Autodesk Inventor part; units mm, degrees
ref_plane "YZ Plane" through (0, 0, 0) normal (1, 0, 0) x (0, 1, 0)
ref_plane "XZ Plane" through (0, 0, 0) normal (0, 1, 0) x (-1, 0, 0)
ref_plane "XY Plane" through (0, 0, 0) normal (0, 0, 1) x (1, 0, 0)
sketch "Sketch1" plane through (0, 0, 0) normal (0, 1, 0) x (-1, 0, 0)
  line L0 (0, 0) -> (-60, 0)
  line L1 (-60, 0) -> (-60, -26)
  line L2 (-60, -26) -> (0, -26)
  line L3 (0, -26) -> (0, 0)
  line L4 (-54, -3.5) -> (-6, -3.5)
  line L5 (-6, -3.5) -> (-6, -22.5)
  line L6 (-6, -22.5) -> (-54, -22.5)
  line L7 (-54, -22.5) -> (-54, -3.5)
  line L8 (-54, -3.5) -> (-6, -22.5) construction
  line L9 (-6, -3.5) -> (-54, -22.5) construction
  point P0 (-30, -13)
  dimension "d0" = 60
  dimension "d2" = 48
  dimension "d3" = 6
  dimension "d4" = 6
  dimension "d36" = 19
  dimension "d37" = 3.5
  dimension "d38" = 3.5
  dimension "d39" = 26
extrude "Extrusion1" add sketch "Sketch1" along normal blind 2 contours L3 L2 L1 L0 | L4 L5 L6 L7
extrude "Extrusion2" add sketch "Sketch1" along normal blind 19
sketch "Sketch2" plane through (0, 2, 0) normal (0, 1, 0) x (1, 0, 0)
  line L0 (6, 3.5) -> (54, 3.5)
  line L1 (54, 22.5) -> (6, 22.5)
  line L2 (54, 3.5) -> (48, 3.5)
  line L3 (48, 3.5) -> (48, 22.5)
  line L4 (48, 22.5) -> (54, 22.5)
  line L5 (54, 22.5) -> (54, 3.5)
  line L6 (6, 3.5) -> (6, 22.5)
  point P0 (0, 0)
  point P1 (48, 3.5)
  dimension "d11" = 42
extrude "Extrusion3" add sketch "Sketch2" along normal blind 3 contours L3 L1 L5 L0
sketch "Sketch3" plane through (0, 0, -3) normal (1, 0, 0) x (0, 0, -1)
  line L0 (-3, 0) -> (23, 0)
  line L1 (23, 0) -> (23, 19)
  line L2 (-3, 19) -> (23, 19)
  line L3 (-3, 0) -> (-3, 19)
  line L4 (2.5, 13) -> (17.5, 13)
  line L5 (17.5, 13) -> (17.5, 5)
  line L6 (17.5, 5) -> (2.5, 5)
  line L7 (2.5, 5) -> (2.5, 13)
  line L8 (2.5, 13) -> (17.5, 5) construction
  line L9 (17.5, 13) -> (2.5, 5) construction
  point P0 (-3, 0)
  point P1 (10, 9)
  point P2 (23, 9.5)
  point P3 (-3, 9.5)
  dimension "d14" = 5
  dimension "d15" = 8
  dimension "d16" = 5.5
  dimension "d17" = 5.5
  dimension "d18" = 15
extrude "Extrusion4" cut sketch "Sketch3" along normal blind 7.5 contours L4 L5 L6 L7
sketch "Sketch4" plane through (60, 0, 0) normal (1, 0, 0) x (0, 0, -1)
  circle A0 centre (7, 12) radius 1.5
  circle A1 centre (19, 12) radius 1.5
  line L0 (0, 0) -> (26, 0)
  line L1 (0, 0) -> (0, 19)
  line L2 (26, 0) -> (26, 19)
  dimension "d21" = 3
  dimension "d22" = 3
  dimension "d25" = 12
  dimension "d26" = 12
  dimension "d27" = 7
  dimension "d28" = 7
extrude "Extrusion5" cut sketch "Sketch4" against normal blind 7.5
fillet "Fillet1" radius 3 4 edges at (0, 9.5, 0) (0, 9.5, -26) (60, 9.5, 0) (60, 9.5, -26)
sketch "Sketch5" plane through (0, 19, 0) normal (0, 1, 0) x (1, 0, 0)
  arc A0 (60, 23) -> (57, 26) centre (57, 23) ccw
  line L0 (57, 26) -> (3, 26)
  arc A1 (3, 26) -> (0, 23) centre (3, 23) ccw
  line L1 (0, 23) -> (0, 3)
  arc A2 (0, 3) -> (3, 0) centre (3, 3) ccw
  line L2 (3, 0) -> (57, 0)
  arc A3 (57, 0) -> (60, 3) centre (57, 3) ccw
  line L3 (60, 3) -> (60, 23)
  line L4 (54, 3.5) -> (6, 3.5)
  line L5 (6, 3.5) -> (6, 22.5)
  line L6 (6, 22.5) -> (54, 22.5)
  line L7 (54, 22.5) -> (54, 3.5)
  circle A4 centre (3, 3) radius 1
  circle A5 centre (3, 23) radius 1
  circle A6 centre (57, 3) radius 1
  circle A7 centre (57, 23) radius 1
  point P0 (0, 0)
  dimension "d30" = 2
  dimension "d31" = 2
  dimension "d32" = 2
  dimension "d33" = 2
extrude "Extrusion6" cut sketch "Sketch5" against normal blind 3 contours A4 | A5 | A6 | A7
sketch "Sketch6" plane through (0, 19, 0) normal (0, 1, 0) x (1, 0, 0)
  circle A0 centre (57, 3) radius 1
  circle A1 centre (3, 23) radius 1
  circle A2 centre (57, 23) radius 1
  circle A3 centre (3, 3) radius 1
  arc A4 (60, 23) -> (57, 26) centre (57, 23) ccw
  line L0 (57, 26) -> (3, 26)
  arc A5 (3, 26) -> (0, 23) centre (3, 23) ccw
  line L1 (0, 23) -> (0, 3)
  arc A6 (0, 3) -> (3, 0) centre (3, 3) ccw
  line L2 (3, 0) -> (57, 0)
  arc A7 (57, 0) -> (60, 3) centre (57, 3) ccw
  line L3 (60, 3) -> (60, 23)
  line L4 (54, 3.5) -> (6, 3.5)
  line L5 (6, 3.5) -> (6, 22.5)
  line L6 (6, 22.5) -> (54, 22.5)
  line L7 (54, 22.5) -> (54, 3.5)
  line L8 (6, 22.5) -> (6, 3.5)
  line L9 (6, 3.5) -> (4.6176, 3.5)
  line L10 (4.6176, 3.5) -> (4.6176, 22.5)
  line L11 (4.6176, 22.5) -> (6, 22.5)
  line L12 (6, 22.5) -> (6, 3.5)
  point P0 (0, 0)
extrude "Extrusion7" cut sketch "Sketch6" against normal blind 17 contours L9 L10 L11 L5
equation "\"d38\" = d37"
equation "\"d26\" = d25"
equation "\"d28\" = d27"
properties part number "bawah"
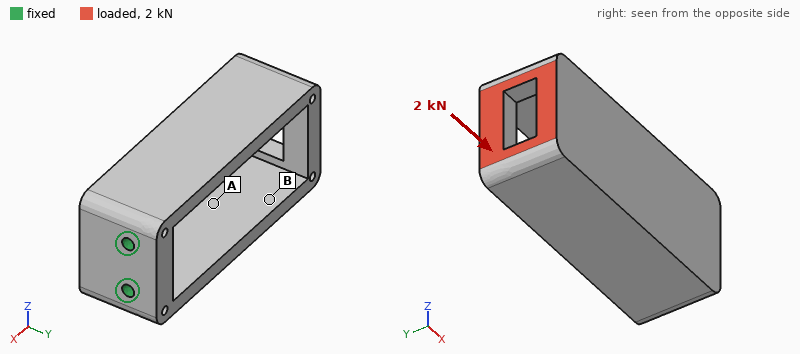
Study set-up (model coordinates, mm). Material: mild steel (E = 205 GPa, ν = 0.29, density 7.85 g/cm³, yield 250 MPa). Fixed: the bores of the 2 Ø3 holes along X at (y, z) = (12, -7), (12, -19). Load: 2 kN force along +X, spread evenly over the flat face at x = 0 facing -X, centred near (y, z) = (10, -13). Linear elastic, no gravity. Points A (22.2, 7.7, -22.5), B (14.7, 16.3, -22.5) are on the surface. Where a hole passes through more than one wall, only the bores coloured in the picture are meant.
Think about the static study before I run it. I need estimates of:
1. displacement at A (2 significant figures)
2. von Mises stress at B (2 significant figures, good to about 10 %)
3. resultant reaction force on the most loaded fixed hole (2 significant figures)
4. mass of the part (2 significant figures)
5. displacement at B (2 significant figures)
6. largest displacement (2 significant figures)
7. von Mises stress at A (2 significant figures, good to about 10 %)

4.6 µm
31 MPa
1.0 kN
100 g
7.5 µm
16 µm
13 MPa
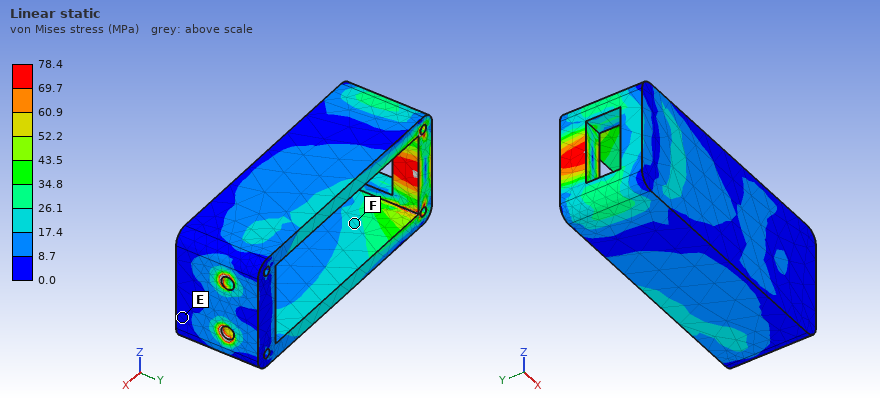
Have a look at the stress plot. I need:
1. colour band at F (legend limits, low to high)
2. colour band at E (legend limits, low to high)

17.4 to 26.1 MPa
0.0 to 8.7 MPa
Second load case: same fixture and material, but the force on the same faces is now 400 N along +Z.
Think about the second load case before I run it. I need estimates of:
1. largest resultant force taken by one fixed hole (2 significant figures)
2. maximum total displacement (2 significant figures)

1.2 kN
95 µm
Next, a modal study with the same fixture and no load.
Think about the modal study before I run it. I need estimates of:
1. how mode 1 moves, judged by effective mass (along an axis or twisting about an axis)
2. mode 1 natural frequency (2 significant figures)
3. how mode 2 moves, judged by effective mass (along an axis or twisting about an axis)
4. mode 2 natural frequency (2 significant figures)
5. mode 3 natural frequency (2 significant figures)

along Z
2000 Hz
along Y
2200 Hz
6600 Hz
